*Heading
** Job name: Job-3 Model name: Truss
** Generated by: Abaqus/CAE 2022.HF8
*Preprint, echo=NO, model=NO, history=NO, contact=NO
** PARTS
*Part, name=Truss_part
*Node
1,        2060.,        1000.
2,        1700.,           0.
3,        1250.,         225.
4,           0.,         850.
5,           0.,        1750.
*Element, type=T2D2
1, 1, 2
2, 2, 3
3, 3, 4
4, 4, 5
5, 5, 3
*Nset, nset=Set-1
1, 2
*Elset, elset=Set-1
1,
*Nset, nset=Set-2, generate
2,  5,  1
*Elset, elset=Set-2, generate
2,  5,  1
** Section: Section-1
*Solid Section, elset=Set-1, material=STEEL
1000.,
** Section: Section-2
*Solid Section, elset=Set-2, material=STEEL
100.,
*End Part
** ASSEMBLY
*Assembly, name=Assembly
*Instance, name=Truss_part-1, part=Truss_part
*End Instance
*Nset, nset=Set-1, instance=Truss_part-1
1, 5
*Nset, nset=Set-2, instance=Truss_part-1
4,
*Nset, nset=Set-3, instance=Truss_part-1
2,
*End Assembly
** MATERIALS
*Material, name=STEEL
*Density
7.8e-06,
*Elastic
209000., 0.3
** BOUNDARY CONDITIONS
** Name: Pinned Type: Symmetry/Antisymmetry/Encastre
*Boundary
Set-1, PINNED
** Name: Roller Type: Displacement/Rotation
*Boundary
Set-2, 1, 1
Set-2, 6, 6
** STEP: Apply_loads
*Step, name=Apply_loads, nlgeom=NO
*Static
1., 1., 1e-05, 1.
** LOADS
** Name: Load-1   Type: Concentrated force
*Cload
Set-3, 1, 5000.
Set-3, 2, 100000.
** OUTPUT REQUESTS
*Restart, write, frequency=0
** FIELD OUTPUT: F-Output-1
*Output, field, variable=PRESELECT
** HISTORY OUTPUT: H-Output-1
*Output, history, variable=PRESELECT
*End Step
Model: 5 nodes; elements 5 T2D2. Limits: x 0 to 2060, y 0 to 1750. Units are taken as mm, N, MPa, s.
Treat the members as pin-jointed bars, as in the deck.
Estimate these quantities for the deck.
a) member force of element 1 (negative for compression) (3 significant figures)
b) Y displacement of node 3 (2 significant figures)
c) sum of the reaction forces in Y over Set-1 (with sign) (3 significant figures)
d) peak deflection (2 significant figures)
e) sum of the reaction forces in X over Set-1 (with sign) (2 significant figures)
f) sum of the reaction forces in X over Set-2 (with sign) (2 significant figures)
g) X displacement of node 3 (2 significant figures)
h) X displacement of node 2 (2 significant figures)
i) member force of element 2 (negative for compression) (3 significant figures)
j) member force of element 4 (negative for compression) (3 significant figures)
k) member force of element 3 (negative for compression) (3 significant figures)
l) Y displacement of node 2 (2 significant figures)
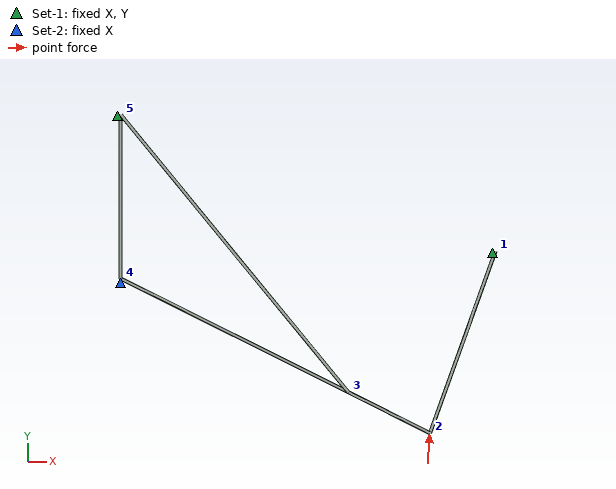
-92300 N
-3.4 mm
-1.00e+05 N
5.4 mm
-31000 N
26000 N
-4.2 mm
-2.6 mm
-29400 N
-13100 N
-29400 N
1.4 mm
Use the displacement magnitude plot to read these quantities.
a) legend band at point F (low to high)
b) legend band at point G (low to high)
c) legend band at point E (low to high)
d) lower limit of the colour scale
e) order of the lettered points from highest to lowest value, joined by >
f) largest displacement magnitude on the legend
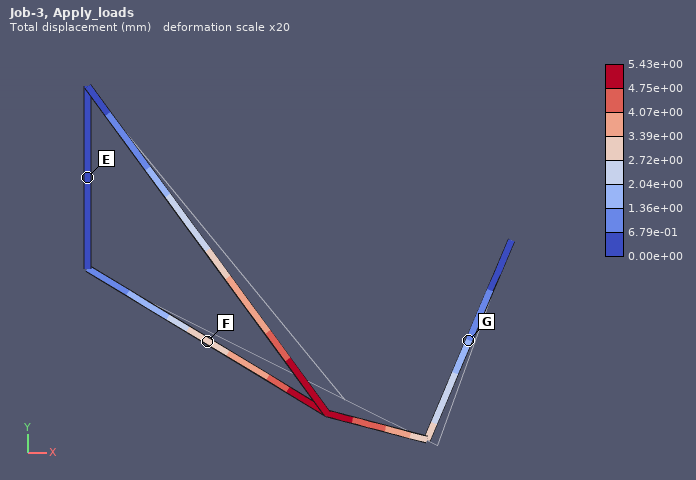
2.72e+00 to 3.39e+00 mm
1.36e+00 to 2.04e+00 mm
0.00e+00 to 6.79e-01 mm
0.00e+00 mm
F > G > E
5.43e+00 mm
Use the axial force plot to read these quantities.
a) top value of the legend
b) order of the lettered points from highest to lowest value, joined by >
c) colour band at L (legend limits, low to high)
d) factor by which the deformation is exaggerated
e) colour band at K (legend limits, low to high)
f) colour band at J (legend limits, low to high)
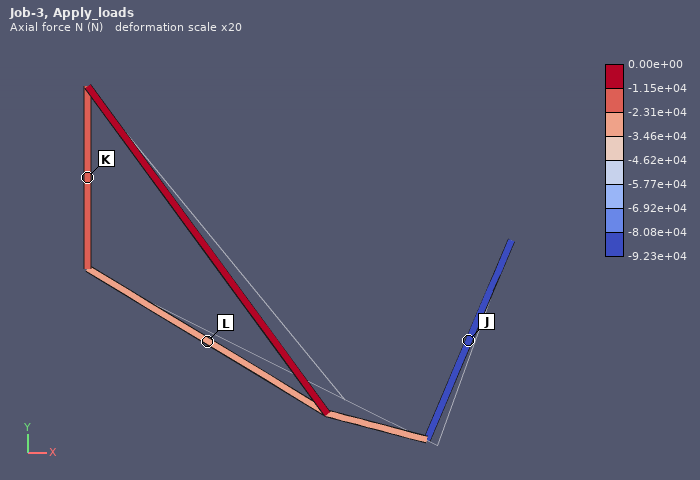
0.00e+00 N
K > L > J
-3.46e+04 to -2.31e+04 N
20
-2.31e+04 to -1.15e+04 N
-9.23e+04 to -8.08e+04 N
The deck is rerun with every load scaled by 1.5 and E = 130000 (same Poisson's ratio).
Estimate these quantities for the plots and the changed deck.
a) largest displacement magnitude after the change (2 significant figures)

13 mm
